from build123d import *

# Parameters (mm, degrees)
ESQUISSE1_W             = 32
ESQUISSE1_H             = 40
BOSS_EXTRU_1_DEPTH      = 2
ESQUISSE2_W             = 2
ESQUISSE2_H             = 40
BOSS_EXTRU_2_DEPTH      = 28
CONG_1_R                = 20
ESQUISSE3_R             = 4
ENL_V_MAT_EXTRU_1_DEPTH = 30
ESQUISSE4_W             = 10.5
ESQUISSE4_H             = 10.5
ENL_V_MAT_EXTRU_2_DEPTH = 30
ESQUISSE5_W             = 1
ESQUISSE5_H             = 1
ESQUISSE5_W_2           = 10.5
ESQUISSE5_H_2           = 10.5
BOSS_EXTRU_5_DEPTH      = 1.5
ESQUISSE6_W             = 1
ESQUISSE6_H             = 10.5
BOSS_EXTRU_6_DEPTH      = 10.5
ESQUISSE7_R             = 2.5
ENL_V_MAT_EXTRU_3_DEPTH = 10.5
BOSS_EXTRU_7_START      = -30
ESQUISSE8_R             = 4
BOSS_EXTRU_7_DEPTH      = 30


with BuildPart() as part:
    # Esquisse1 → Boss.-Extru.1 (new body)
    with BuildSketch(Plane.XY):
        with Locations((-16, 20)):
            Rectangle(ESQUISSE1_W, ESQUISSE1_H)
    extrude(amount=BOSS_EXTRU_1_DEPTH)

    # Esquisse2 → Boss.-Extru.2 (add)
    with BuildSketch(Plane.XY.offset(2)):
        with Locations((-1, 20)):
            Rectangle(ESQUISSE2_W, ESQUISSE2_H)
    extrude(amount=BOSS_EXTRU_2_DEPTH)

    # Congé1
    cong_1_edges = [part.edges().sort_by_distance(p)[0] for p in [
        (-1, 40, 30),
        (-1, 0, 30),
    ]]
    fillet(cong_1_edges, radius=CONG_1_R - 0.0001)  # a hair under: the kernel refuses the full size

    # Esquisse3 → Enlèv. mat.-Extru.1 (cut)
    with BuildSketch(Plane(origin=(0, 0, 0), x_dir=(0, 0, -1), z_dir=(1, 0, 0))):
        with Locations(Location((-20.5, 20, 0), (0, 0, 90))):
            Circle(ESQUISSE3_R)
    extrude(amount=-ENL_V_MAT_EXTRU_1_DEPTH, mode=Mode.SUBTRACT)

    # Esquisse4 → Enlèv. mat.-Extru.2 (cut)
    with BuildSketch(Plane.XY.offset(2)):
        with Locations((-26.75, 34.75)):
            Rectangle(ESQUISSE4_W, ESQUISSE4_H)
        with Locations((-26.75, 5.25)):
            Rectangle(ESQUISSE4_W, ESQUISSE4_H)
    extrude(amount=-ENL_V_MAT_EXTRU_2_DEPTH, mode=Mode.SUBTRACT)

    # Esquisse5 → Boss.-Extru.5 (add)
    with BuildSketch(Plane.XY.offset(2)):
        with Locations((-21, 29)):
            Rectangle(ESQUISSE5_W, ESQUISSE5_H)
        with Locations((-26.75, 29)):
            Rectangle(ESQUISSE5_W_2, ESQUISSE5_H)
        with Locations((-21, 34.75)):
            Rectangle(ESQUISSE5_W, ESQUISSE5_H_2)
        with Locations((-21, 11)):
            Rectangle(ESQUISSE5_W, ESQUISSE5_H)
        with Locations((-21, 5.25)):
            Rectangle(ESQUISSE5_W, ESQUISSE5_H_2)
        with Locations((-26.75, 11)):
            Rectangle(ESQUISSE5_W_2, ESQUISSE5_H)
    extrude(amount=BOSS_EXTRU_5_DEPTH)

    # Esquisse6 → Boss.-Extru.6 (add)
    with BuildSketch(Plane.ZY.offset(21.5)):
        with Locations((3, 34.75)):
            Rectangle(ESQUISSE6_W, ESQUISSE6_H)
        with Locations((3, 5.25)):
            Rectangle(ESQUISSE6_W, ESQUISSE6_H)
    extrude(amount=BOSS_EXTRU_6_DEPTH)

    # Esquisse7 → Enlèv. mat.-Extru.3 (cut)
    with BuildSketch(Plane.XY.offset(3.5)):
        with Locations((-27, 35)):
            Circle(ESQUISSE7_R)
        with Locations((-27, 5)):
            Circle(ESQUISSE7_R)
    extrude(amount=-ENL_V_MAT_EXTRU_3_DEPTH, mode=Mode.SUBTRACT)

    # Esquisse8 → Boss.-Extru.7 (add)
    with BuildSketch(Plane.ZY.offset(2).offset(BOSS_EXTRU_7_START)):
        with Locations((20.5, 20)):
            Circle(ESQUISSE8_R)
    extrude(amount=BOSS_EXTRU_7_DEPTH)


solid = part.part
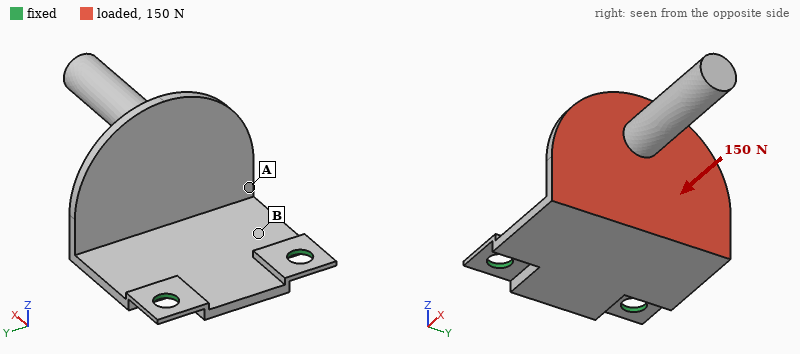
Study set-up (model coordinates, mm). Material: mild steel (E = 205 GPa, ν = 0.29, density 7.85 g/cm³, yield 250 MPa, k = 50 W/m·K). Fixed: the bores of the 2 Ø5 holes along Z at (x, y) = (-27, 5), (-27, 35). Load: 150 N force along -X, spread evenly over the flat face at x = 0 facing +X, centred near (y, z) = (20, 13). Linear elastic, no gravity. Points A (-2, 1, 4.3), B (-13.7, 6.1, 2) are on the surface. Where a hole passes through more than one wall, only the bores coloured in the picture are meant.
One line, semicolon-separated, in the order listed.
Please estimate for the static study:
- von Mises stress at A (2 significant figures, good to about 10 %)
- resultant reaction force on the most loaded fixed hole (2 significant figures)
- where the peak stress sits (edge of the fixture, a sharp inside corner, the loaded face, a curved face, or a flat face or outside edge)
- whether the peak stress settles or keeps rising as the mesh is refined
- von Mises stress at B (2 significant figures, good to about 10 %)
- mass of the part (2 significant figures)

35 MPa; 89 N; edge of the fixture; keeps rising; 66 MPa; 45 g
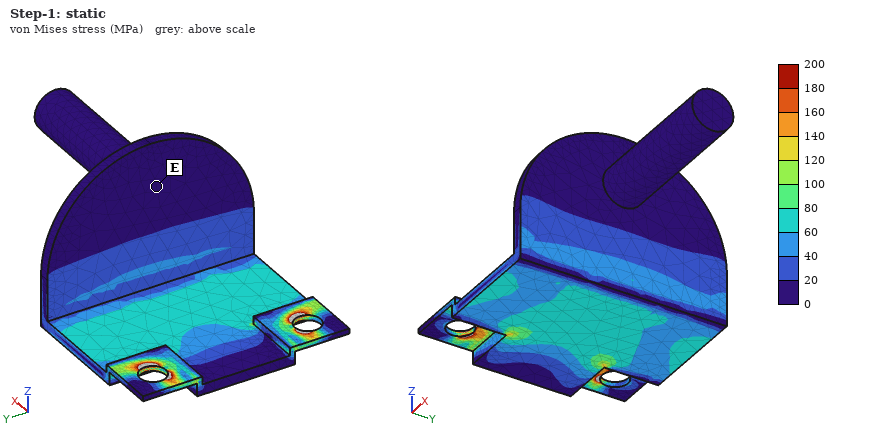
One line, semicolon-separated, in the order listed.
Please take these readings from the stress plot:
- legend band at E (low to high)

0 to 20 MPa
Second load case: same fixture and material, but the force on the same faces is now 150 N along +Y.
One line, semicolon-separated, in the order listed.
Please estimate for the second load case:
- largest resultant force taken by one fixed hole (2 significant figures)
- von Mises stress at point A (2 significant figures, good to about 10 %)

150 N; 37 MPa
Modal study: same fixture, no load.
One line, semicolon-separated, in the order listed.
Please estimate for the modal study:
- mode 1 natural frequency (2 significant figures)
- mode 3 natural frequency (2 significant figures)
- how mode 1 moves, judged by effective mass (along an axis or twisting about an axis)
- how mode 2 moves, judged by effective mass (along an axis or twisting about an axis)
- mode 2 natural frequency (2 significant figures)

380 Hz; 1500 Hz; along Z; along Y; 1100 Hz
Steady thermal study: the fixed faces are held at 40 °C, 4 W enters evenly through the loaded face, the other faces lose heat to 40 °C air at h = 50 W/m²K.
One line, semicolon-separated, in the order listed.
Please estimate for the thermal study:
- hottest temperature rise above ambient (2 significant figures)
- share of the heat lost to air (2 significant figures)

20 K; 65 %
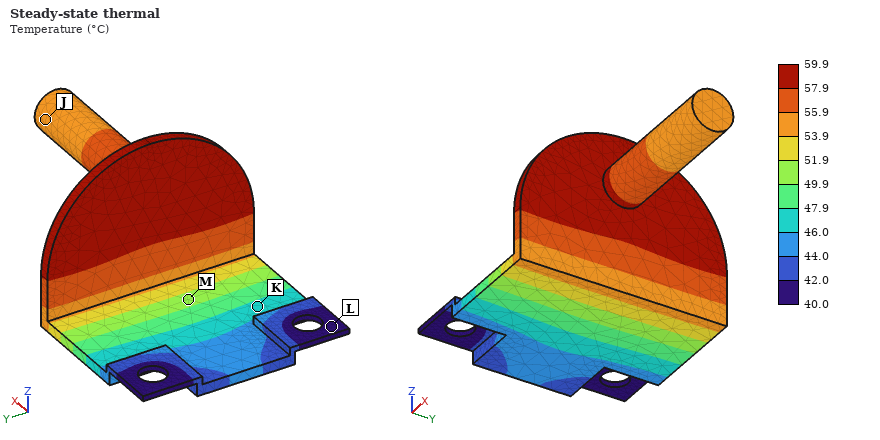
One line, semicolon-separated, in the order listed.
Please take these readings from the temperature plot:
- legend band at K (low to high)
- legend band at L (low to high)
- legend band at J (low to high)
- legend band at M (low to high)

46.0 to 47.9 °C; 40.0 to 42.0 °C; 53.9 to 55.9 °C; 49.9 to 51.9 °C
